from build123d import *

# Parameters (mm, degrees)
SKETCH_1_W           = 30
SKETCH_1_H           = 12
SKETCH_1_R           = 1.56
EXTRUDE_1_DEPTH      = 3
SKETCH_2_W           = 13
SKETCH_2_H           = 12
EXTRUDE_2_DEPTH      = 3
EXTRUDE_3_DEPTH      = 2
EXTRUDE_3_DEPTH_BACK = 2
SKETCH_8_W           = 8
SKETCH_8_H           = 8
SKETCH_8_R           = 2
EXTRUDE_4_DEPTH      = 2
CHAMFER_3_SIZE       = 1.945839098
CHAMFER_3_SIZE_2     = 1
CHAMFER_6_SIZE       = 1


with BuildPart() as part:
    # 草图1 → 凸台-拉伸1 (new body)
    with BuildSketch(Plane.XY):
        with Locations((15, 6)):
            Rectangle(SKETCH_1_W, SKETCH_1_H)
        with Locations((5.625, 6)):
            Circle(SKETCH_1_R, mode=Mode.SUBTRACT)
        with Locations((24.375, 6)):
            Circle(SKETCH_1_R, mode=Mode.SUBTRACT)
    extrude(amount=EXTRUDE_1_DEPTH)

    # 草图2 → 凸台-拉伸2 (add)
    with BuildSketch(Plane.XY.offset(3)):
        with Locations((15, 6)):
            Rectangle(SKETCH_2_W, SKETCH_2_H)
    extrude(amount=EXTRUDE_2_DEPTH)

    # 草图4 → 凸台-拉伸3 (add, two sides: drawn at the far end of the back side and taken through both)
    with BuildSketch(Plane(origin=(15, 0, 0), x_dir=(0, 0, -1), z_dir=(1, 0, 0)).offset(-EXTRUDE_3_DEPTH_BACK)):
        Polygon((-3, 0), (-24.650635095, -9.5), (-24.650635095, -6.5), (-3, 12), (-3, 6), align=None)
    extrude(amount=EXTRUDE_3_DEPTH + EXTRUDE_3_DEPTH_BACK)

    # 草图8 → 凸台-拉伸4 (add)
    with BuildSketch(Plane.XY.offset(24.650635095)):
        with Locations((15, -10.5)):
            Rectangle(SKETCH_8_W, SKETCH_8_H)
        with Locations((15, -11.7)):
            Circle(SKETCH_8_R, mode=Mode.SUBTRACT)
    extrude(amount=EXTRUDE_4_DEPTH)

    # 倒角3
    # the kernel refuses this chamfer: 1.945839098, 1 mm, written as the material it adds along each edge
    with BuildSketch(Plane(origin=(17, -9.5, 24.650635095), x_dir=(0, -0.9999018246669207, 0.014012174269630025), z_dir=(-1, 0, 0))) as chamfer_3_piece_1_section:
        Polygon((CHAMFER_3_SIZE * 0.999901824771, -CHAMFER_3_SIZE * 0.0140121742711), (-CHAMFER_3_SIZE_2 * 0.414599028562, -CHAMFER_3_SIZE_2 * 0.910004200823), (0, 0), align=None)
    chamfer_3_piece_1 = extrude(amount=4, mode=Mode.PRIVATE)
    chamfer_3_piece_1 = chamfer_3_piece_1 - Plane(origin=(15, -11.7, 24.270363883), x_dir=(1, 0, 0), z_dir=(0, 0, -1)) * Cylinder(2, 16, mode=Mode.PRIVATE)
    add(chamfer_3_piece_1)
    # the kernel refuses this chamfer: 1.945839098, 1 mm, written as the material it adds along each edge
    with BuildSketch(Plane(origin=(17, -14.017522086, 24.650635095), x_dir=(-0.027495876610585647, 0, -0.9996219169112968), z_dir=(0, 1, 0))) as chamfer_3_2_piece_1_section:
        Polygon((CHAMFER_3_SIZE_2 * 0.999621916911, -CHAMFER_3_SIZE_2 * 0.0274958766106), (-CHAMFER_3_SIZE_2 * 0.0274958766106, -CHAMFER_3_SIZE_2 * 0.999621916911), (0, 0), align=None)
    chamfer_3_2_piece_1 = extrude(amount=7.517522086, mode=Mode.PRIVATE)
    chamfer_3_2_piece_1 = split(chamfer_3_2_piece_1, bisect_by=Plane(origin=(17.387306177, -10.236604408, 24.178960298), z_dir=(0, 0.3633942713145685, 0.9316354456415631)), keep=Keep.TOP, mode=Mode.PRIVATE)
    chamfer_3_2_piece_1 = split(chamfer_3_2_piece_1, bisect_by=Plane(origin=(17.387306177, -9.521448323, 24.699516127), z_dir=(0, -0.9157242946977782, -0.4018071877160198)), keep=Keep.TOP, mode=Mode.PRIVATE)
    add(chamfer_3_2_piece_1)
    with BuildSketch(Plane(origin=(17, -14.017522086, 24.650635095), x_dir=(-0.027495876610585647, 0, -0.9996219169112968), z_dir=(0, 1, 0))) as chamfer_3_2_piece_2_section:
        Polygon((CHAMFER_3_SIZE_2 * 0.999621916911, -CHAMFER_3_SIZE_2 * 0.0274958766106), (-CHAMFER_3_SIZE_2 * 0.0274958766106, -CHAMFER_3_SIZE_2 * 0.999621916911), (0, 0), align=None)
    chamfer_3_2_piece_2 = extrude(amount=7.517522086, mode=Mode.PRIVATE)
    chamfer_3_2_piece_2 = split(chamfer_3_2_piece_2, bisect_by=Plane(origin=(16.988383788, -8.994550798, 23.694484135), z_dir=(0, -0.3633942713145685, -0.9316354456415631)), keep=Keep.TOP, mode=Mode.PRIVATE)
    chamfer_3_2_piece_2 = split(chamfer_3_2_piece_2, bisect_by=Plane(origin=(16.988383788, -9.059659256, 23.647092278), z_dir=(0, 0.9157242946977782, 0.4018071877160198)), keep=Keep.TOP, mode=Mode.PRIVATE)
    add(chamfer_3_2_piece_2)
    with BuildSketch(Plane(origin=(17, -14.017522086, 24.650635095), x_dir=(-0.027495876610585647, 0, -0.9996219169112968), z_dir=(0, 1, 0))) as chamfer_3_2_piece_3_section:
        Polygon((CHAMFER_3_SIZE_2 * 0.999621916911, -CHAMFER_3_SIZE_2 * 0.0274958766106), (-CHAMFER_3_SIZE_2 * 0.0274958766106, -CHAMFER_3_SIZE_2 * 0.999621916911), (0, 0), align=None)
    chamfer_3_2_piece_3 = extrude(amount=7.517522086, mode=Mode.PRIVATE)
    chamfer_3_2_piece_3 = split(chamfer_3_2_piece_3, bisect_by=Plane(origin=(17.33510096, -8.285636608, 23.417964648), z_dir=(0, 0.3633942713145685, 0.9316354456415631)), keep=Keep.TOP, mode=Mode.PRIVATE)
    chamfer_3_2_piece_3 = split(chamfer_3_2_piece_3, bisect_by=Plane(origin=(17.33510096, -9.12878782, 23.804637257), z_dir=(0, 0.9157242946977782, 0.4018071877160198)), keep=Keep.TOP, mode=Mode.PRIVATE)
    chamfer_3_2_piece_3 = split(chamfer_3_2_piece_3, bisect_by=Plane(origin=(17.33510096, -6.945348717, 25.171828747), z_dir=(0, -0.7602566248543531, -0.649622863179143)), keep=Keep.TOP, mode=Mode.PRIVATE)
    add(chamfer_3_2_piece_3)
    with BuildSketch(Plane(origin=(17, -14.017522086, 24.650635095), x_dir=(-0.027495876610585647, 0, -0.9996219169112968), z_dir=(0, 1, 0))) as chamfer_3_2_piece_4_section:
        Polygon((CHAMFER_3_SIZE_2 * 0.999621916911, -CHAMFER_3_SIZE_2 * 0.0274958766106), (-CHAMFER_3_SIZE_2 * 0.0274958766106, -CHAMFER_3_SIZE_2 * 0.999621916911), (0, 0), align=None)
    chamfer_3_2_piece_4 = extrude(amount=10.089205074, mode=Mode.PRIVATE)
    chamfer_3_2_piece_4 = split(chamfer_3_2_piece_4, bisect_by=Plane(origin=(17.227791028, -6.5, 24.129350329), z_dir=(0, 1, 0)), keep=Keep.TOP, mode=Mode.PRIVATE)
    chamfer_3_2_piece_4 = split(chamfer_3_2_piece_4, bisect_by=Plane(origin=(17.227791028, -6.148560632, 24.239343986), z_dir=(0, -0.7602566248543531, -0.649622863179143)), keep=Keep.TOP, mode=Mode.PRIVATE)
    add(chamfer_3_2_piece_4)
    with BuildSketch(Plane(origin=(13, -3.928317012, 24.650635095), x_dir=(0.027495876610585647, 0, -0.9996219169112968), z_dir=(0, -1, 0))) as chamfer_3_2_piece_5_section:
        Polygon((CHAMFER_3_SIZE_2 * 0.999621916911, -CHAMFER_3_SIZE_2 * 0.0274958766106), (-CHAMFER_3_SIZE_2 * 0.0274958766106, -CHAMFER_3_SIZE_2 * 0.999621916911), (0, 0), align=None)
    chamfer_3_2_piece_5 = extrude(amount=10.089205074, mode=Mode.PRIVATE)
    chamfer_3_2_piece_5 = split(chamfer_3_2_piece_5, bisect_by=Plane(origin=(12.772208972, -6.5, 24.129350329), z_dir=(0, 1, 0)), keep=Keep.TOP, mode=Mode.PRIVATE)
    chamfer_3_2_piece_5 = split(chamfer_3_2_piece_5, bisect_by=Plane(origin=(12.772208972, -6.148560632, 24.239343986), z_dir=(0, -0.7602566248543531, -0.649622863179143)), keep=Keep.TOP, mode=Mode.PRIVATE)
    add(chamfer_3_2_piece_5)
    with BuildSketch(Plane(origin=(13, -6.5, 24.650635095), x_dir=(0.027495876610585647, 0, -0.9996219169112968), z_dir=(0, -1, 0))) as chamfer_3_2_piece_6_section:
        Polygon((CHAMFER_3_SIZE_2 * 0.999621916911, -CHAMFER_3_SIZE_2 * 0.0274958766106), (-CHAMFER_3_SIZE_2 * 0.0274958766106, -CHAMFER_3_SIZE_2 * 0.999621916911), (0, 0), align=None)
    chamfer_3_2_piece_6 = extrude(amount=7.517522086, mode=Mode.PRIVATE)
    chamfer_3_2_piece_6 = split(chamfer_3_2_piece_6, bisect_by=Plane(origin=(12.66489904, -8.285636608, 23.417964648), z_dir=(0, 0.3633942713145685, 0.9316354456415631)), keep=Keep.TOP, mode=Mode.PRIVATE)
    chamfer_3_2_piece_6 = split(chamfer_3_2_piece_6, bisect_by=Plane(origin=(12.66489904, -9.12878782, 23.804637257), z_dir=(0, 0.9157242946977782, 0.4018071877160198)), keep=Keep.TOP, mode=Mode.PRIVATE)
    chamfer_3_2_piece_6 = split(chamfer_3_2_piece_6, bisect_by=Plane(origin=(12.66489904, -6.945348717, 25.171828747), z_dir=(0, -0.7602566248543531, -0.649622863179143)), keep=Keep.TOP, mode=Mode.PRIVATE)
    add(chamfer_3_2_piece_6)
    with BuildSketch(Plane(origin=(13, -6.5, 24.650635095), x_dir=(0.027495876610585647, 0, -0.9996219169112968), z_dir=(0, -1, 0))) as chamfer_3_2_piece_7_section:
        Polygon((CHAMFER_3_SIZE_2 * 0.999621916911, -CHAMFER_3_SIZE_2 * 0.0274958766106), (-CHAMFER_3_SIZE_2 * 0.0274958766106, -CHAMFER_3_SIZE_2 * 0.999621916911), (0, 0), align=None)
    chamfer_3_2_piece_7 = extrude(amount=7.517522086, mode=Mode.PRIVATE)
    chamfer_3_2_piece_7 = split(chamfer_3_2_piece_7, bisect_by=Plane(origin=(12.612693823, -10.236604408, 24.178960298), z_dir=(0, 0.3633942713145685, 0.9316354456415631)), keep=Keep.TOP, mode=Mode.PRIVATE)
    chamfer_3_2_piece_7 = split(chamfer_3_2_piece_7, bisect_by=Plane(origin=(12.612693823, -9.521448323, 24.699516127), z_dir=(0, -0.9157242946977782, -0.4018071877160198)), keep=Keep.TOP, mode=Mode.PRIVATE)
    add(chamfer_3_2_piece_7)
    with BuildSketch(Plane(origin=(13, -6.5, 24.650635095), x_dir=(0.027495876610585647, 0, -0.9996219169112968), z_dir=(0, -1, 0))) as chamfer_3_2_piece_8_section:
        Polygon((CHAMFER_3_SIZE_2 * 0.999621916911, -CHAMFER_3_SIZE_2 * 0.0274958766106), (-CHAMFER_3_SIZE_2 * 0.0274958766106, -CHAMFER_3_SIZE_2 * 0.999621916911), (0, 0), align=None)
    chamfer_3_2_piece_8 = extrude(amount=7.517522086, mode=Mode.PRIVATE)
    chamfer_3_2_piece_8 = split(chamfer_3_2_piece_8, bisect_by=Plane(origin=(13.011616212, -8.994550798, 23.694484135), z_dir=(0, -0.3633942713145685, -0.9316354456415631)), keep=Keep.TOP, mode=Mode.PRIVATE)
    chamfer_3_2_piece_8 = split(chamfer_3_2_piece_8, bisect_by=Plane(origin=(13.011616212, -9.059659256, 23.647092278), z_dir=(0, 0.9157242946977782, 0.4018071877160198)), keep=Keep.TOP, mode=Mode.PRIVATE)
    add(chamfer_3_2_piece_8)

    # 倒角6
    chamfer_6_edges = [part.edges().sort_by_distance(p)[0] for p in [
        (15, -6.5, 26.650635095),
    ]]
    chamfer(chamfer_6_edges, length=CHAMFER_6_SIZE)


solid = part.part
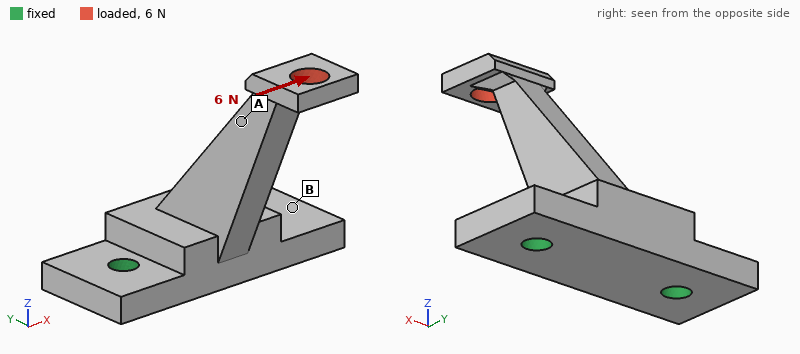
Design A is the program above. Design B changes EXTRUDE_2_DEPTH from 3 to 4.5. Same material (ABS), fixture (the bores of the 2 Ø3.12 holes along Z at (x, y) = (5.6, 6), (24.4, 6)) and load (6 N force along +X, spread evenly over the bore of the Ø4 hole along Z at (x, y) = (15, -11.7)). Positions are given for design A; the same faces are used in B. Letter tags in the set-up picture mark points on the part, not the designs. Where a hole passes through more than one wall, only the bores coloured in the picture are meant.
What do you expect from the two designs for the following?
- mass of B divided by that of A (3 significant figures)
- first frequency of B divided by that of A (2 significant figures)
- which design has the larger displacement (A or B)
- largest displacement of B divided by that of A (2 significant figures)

1.09
1.1
A
0.89
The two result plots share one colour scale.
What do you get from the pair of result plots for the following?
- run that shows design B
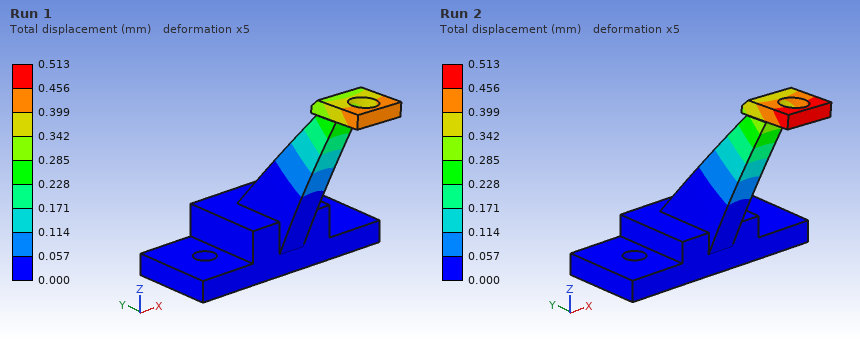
Run 1
